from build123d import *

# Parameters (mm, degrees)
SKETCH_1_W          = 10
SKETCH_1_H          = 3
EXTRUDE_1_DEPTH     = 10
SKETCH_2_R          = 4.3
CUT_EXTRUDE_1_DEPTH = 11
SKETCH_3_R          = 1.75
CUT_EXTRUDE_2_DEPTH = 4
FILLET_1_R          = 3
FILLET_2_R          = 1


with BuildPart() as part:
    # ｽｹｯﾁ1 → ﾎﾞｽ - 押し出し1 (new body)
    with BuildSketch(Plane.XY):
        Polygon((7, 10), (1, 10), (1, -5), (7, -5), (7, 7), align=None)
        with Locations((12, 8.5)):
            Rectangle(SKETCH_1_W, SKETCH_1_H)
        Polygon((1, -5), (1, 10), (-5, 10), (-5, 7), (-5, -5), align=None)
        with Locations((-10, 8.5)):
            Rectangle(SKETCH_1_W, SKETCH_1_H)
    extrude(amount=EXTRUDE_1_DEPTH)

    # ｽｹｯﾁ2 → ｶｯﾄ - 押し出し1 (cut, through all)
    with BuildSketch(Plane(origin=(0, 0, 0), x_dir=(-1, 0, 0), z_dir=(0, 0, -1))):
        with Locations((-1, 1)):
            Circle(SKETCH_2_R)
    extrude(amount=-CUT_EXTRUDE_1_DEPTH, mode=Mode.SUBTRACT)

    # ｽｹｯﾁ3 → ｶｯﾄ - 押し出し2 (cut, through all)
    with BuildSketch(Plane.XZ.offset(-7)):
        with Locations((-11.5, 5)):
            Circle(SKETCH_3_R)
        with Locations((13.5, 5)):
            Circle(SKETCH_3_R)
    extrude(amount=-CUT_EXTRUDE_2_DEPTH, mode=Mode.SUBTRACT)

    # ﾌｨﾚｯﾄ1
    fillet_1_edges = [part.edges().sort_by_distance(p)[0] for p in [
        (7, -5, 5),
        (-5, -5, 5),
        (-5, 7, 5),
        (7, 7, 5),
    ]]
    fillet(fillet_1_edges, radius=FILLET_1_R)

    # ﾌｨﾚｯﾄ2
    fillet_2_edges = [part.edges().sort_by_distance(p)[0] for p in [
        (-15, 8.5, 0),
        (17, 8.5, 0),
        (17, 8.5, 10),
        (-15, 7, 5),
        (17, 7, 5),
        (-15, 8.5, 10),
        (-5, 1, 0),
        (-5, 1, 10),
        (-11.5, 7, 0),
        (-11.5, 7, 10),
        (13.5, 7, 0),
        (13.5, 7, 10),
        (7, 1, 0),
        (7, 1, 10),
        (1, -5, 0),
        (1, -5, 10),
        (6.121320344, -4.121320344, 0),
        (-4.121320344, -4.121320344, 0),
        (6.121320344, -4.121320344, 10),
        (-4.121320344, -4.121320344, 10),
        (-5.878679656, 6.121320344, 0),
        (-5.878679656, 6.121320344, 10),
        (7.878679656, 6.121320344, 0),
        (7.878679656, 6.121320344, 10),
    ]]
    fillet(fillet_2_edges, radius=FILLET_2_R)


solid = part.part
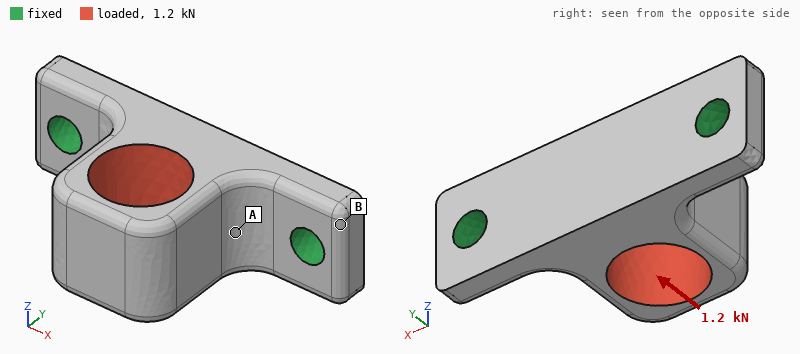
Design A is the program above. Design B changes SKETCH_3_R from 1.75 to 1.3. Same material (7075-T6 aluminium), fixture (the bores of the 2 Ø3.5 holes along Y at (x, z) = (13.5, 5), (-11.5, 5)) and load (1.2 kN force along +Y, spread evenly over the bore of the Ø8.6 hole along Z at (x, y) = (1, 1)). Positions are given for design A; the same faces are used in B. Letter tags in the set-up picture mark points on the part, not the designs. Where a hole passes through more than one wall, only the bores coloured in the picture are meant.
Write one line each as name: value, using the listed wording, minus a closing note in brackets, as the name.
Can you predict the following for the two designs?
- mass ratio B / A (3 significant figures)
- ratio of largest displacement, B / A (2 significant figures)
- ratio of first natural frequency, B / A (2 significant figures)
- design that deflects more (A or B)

mass ratio B / A: 1.01
ratio of largest displacement, B / A: 1.2
ratio of first natural frequency, B / A: 0.91
design that deflects more: B
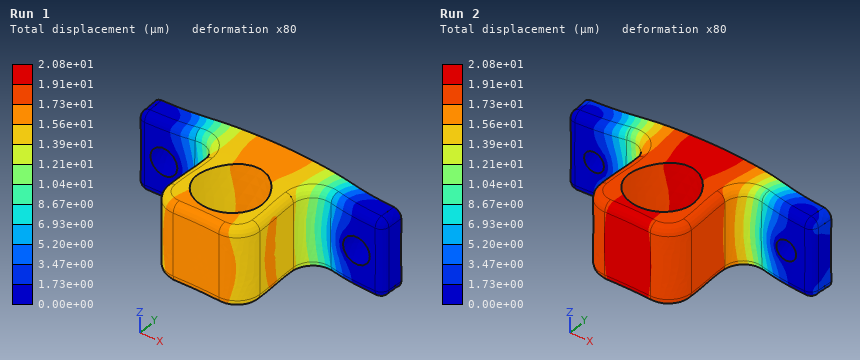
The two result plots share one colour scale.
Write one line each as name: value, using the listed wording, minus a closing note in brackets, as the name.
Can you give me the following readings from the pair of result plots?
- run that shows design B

run that shows design B: Run 2
